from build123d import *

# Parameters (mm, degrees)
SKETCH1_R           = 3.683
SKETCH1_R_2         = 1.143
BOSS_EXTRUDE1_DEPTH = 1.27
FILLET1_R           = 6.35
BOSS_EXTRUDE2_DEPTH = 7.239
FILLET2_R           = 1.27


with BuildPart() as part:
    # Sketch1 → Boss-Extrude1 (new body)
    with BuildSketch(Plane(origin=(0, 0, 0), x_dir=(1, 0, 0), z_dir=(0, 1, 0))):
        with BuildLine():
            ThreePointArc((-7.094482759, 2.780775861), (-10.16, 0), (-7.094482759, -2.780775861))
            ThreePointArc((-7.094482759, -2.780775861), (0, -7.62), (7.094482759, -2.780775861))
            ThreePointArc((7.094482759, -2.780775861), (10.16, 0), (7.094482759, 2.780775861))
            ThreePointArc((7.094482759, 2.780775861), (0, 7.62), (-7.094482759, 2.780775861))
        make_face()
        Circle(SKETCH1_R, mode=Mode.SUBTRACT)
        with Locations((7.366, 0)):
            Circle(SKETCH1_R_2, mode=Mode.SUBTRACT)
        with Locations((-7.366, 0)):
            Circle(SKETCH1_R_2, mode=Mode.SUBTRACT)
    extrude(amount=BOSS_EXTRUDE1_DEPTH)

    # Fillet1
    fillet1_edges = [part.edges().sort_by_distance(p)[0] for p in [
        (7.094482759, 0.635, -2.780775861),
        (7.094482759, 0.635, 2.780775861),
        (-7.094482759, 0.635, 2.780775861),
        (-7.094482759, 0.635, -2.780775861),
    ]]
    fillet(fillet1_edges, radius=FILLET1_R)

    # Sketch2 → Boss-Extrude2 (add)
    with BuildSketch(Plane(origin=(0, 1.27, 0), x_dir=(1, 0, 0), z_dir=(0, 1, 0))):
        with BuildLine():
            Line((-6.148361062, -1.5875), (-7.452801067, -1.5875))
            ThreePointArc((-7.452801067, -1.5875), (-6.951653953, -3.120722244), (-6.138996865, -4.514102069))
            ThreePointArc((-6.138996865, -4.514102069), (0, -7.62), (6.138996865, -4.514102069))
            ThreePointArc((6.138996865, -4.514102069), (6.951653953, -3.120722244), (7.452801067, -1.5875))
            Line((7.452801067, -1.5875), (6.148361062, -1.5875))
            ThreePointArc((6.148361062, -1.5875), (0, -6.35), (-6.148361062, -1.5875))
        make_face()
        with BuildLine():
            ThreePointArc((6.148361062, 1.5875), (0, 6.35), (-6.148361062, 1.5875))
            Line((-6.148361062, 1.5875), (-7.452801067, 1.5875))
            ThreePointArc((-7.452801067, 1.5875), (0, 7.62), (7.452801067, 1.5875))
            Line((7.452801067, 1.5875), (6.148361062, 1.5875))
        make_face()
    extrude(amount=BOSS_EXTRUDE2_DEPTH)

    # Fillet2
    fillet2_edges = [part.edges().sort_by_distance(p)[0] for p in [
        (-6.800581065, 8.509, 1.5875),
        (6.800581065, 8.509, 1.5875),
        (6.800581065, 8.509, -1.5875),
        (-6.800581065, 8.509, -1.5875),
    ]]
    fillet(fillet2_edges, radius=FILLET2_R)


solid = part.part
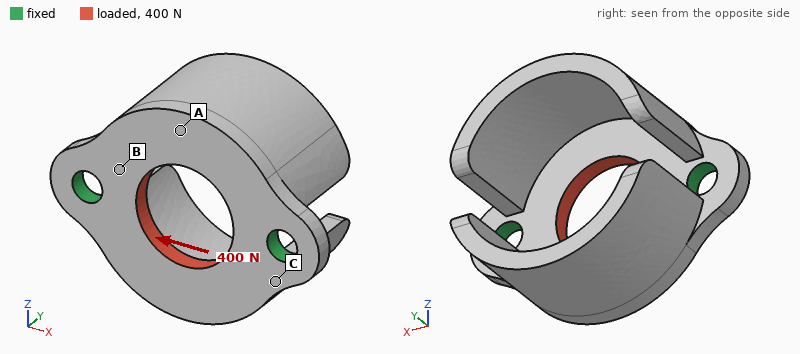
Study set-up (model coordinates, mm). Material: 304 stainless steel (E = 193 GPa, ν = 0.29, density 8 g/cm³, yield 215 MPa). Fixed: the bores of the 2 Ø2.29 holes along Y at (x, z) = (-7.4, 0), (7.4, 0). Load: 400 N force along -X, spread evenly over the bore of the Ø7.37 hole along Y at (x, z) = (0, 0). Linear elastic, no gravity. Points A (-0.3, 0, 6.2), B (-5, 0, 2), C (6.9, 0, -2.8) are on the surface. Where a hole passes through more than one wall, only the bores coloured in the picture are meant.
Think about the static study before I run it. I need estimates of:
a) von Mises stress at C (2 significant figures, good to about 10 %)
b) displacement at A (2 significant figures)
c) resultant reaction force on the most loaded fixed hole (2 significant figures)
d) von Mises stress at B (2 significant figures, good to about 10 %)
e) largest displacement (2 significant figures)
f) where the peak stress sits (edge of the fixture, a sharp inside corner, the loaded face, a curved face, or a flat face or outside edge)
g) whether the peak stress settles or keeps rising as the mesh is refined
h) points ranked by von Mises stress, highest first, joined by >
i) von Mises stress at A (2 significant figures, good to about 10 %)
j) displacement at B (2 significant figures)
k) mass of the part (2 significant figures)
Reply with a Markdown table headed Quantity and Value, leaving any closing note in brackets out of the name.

| Quantity | Value |
|---|---|
| von Mises stress at C | 17 MPa |
| displacement at A | 0.69 µm |
| resultant reaction force on the most loaded fixed hole | 200 N |
| von Mises stress at B | 29 MPa |
| largest displacement | 1.0 µm |
| where the peak stress sits | edge of the fixture |
| whether the peak stress settles or keeps rising as the mesh is refined | keeps rising |
| points ranked by von Mises stress, highest first, joined by > | B > C > A |
| von Mises stress at A | 7.5 MPa |
| displacement at B | 0.43 µm |
| mass of the part | 4.3 g |
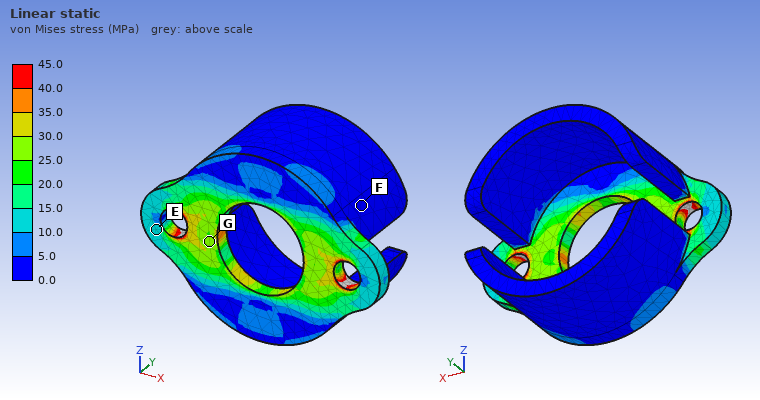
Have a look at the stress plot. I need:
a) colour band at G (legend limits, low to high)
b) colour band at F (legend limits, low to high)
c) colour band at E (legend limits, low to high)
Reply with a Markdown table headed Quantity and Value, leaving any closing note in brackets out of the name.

| Quantity | Value |
|---|---|
| colour band at G | 25.0 to 30.0 MPa |
| colour band at F | 0.0 to 5.0 MPa |
| colour band at E | 10.0 to 15.0 MPa |
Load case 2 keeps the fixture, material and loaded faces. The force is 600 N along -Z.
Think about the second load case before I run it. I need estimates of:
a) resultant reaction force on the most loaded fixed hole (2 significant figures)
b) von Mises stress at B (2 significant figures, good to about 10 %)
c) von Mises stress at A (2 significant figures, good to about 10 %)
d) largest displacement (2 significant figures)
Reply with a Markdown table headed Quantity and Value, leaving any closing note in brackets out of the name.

| Quantity | Value |
|---|---|
| resultant reaction force on the most loaded fixed hole | 300 N |
| von Mises stress at B | 37 MPa |
| von Mises stress at A | 26 MPa |
| largest displacement | 2.1 µm |
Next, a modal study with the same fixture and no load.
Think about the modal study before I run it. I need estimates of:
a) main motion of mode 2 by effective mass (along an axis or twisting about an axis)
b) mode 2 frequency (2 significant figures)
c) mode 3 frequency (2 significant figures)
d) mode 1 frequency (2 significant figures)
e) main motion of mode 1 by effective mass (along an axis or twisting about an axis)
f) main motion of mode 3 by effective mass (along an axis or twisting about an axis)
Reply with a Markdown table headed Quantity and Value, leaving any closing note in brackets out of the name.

| Quantity | Value |
|---|---|
| main motion of mode 2 by effective mass | along Y |
| mode 2 frequency | 7900 Hz |
| mode 3 frequency | 17 kHz |
| mode 1 frequency | 7400 Hz |
| main motion of mode 1 by effective mass | along Z |
| main motion of mode 3 by effective mass | along X |
